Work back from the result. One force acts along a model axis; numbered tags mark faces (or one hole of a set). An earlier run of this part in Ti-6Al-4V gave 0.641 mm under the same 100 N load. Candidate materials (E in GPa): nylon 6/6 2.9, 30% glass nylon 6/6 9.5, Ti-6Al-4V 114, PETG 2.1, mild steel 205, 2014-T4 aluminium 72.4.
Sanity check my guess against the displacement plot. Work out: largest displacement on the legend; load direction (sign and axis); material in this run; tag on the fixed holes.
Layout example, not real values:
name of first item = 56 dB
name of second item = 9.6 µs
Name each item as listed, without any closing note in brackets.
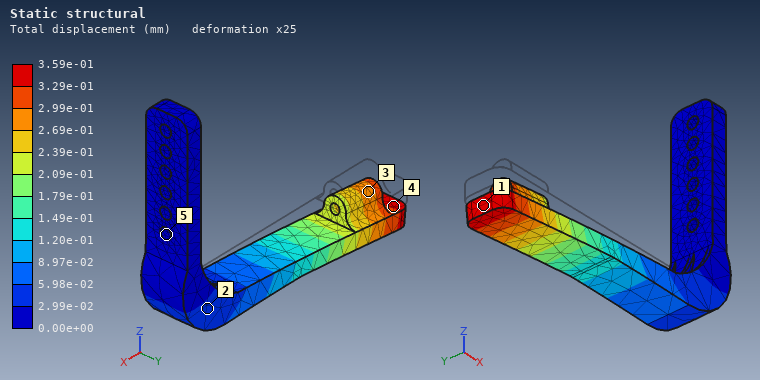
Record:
largest displacement on the legend = 3.59e-01 mm
load direction = -Z
material in this run = mild steel
tag on the fixed holes = 5
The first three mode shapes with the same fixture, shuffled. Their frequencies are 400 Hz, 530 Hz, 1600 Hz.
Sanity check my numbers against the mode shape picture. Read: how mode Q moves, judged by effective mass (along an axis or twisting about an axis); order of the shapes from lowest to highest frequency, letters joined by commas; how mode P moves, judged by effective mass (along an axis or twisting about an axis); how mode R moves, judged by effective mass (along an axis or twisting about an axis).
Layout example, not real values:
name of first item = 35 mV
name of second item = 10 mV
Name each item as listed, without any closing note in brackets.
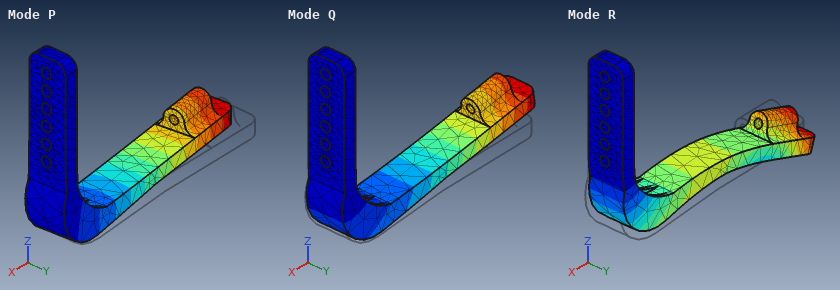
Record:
how mode Q moves, judged by effective mass = along Z
order of the shapes from lowest to highest frequency, letters joined by commas = Q, P, R
how mode P moves, judged by effective mass = along Y
how mode R moves, judged by effective mass = along X
